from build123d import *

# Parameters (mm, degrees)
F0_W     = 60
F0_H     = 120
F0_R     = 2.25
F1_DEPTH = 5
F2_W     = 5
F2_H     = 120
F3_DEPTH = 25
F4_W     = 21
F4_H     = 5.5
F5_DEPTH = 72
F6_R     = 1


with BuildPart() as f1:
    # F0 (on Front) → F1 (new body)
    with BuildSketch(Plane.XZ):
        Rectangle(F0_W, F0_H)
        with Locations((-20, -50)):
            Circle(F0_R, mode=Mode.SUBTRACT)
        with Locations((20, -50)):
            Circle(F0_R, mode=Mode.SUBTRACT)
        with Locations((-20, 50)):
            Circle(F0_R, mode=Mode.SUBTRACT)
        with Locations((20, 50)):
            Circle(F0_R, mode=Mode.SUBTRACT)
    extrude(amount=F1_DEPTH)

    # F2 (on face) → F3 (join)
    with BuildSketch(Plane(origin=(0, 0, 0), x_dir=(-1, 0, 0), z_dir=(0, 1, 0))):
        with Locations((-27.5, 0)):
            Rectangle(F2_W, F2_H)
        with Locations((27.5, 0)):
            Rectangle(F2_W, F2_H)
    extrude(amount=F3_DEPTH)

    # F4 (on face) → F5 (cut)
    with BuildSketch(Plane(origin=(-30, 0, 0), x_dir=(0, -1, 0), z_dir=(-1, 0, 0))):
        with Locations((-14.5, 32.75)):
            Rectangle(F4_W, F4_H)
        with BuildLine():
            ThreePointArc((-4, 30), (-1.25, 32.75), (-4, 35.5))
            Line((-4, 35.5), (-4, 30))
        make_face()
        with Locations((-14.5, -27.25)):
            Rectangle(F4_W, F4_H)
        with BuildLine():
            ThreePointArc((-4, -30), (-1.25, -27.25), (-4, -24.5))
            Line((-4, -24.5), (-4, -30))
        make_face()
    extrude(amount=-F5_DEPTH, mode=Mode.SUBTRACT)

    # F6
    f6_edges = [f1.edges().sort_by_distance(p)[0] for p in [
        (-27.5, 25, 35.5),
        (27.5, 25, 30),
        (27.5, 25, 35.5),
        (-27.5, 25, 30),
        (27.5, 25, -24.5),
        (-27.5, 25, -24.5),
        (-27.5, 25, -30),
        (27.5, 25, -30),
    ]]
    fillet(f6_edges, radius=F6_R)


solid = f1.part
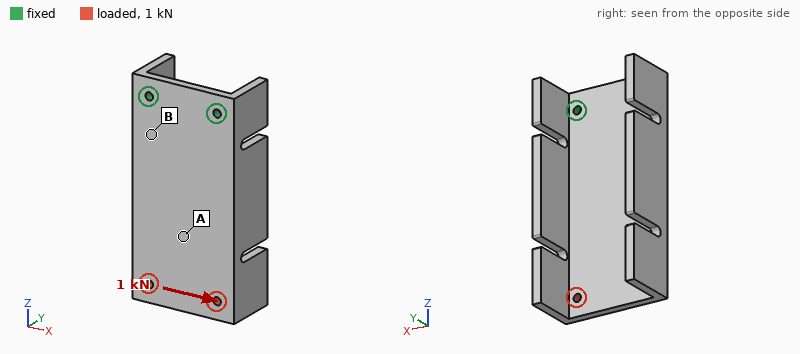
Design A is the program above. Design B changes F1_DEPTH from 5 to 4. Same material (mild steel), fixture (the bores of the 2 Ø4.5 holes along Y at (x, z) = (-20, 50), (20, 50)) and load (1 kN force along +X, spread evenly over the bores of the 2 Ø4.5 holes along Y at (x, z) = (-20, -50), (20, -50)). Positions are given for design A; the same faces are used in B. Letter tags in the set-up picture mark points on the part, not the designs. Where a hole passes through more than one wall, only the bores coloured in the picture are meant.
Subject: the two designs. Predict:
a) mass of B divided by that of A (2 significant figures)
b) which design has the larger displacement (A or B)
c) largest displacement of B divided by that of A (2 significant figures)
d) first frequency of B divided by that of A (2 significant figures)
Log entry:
0.89
B
1.2
0.83
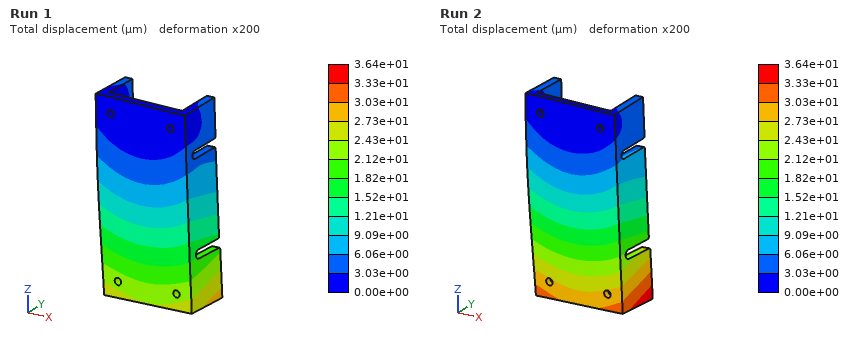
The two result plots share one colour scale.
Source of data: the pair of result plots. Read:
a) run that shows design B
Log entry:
Run 2
